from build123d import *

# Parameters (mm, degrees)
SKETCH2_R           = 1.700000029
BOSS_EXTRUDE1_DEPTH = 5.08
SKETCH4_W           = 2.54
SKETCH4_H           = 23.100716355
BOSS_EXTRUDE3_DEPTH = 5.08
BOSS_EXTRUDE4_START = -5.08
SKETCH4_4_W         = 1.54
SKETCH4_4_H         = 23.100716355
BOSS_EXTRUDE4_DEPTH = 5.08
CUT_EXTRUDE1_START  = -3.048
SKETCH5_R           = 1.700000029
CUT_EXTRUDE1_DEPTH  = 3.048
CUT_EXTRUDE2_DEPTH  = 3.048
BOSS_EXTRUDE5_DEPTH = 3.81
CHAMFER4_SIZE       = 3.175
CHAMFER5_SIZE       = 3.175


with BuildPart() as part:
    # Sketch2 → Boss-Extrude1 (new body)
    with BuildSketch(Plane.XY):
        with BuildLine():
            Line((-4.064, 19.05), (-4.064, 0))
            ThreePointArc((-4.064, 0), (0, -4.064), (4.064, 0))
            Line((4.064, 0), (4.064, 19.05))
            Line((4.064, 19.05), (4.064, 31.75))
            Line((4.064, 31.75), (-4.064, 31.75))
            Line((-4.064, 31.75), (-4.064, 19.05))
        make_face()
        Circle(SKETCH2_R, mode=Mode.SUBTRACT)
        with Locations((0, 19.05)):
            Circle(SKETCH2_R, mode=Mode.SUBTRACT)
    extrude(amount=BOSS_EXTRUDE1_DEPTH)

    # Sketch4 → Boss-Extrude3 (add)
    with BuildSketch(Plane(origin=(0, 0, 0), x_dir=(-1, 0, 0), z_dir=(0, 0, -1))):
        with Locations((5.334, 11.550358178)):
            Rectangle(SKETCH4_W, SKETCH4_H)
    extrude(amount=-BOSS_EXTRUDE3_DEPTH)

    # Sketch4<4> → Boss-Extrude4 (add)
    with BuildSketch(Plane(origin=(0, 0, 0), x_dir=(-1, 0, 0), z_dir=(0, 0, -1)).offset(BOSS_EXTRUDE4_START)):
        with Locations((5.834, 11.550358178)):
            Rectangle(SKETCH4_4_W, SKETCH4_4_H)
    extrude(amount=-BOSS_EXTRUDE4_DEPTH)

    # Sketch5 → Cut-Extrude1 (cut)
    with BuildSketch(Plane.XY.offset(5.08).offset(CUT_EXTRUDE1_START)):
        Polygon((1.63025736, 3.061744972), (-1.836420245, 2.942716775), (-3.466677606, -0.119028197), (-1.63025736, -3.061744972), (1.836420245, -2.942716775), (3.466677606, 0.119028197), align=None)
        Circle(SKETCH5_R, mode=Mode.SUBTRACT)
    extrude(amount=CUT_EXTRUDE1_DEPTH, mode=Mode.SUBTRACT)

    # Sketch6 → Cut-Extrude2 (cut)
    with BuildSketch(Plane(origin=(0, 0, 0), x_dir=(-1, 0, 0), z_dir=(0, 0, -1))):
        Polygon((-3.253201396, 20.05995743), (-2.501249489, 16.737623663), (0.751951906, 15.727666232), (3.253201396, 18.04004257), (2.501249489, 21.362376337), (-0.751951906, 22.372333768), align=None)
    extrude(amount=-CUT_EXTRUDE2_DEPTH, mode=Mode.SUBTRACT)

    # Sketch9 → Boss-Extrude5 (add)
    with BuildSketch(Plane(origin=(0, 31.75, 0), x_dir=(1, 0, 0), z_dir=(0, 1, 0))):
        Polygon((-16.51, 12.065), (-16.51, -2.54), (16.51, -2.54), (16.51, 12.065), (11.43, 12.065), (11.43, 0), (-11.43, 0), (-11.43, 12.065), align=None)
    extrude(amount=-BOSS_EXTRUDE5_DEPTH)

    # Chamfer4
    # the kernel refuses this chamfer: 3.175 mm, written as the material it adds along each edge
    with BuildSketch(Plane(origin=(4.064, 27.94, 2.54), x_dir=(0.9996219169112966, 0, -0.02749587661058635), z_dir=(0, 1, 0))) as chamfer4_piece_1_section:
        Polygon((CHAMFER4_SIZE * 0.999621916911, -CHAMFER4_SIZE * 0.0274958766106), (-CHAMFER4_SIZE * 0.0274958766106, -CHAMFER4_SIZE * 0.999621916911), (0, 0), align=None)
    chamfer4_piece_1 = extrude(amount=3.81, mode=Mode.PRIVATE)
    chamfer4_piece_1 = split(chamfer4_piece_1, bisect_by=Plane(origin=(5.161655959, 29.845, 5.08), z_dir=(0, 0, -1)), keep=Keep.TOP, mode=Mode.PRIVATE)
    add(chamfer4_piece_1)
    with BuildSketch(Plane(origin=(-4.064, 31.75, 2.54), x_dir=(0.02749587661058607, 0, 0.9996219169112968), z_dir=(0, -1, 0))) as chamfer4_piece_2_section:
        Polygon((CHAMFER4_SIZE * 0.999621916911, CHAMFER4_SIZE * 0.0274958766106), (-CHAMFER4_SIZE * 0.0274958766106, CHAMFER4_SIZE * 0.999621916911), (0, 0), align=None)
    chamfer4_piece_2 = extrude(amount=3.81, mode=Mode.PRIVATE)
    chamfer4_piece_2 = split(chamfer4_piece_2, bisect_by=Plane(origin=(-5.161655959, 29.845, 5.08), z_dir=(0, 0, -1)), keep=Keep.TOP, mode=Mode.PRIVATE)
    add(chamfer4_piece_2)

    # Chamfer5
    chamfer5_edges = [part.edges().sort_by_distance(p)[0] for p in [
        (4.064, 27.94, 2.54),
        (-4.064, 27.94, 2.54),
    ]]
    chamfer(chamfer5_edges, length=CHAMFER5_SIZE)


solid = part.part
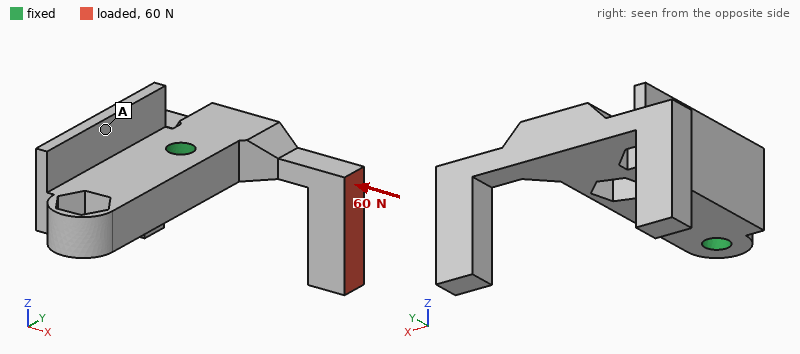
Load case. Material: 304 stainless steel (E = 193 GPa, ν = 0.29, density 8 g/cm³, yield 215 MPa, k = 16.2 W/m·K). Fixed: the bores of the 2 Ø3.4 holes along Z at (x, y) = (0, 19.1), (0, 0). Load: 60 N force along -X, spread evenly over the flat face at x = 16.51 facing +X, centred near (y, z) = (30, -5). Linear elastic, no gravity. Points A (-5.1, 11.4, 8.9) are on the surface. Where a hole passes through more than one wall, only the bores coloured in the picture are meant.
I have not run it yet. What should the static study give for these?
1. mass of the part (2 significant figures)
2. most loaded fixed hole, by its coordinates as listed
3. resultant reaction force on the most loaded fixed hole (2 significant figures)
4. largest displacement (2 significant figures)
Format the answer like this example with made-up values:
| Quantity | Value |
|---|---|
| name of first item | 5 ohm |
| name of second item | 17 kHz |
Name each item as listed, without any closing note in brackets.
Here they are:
| Quantity | Value |
|---|---|
| mass of the part | 20 g |
| most loaded fixed hole, by its coordinates as listed | (0, 19.1) |
| resultant reaction force on the most loaded fixed hole | 77 N |
| largest displacement | 50 µm |
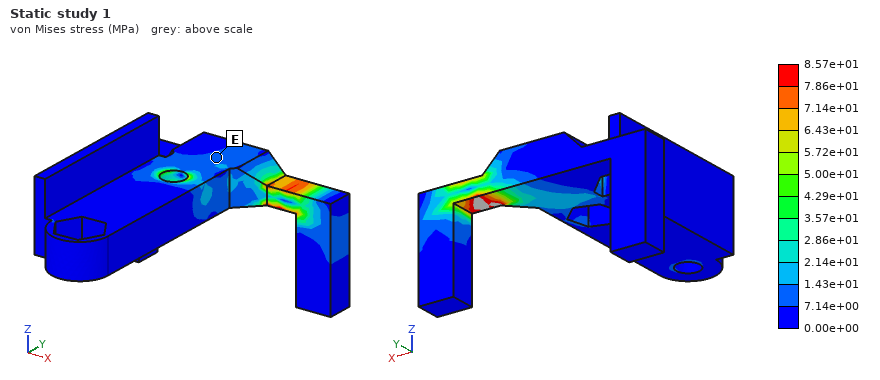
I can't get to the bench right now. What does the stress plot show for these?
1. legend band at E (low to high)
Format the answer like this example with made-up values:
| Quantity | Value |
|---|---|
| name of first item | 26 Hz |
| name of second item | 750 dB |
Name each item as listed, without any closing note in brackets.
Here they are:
| Quantity | Value |
|---|---|
| legend band at E | 7.14e+00 to 1.43e+01 MPa |
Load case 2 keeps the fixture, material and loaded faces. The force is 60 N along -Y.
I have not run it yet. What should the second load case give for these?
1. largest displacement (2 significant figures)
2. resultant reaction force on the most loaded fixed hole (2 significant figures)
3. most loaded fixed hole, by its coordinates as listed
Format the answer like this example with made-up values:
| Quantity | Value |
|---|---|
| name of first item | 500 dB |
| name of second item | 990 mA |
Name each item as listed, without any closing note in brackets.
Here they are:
| Quantity | Value |
|---|---|
| largest displacement | 57 µm |
| resultant reaction force on the most loaded fixed hole | 66 N |
| most loaded fixed hole, by its coordinates as listed | (0, 19.1) |
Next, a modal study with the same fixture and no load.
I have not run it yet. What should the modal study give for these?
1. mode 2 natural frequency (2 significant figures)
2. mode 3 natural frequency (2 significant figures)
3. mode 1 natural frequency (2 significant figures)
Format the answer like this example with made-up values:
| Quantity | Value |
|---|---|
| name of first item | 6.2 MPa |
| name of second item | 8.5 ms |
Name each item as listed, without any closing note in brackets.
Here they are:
| Quantity | Value |
|---|---|
| mode 2 natural frequency | 4000 Hz |
| mode 3 natural frequency | 4400 Hz |
| mode 1 natural frequency | 3300 Hz |
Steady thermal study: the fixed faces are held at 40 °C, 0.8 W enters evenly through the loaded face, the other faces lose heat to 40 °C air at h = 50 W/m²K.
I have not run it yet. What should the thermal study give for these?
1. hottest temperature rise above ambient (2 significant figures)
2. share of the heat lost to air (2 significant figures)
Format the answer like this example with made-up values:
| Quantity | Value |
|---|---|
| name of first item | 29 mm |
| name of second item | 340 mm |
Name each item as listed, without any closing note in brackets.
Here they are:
| Quantity | Value |
|---|---|
| hottest temperature rise above ambient | 35 K |
| share of the heat lost to air | 67 % |
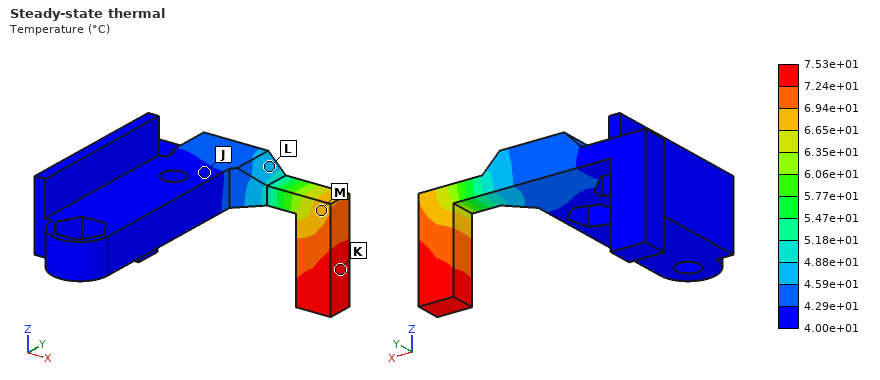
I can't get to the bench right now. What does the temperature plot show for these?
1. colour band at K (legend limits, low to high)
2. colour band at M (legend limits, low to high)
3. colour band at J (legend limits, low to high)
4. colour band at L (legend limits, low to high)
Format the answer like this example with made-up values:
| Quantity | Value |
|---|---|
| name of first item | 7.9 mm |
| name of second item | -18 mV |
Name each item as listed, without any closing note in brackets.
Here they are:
| Quantity | Value |
|---|---|
| colour band at K | 7.24e+01 to 7.53e+01 °C |
| colour band at M | 6.65e+01 to 6.94e+01 °C |
| colour band at J | 4.00e+01 to 4.29e+01 °C |
| colour band at L | 4.59e+01 to 4.88e+01 °C |
